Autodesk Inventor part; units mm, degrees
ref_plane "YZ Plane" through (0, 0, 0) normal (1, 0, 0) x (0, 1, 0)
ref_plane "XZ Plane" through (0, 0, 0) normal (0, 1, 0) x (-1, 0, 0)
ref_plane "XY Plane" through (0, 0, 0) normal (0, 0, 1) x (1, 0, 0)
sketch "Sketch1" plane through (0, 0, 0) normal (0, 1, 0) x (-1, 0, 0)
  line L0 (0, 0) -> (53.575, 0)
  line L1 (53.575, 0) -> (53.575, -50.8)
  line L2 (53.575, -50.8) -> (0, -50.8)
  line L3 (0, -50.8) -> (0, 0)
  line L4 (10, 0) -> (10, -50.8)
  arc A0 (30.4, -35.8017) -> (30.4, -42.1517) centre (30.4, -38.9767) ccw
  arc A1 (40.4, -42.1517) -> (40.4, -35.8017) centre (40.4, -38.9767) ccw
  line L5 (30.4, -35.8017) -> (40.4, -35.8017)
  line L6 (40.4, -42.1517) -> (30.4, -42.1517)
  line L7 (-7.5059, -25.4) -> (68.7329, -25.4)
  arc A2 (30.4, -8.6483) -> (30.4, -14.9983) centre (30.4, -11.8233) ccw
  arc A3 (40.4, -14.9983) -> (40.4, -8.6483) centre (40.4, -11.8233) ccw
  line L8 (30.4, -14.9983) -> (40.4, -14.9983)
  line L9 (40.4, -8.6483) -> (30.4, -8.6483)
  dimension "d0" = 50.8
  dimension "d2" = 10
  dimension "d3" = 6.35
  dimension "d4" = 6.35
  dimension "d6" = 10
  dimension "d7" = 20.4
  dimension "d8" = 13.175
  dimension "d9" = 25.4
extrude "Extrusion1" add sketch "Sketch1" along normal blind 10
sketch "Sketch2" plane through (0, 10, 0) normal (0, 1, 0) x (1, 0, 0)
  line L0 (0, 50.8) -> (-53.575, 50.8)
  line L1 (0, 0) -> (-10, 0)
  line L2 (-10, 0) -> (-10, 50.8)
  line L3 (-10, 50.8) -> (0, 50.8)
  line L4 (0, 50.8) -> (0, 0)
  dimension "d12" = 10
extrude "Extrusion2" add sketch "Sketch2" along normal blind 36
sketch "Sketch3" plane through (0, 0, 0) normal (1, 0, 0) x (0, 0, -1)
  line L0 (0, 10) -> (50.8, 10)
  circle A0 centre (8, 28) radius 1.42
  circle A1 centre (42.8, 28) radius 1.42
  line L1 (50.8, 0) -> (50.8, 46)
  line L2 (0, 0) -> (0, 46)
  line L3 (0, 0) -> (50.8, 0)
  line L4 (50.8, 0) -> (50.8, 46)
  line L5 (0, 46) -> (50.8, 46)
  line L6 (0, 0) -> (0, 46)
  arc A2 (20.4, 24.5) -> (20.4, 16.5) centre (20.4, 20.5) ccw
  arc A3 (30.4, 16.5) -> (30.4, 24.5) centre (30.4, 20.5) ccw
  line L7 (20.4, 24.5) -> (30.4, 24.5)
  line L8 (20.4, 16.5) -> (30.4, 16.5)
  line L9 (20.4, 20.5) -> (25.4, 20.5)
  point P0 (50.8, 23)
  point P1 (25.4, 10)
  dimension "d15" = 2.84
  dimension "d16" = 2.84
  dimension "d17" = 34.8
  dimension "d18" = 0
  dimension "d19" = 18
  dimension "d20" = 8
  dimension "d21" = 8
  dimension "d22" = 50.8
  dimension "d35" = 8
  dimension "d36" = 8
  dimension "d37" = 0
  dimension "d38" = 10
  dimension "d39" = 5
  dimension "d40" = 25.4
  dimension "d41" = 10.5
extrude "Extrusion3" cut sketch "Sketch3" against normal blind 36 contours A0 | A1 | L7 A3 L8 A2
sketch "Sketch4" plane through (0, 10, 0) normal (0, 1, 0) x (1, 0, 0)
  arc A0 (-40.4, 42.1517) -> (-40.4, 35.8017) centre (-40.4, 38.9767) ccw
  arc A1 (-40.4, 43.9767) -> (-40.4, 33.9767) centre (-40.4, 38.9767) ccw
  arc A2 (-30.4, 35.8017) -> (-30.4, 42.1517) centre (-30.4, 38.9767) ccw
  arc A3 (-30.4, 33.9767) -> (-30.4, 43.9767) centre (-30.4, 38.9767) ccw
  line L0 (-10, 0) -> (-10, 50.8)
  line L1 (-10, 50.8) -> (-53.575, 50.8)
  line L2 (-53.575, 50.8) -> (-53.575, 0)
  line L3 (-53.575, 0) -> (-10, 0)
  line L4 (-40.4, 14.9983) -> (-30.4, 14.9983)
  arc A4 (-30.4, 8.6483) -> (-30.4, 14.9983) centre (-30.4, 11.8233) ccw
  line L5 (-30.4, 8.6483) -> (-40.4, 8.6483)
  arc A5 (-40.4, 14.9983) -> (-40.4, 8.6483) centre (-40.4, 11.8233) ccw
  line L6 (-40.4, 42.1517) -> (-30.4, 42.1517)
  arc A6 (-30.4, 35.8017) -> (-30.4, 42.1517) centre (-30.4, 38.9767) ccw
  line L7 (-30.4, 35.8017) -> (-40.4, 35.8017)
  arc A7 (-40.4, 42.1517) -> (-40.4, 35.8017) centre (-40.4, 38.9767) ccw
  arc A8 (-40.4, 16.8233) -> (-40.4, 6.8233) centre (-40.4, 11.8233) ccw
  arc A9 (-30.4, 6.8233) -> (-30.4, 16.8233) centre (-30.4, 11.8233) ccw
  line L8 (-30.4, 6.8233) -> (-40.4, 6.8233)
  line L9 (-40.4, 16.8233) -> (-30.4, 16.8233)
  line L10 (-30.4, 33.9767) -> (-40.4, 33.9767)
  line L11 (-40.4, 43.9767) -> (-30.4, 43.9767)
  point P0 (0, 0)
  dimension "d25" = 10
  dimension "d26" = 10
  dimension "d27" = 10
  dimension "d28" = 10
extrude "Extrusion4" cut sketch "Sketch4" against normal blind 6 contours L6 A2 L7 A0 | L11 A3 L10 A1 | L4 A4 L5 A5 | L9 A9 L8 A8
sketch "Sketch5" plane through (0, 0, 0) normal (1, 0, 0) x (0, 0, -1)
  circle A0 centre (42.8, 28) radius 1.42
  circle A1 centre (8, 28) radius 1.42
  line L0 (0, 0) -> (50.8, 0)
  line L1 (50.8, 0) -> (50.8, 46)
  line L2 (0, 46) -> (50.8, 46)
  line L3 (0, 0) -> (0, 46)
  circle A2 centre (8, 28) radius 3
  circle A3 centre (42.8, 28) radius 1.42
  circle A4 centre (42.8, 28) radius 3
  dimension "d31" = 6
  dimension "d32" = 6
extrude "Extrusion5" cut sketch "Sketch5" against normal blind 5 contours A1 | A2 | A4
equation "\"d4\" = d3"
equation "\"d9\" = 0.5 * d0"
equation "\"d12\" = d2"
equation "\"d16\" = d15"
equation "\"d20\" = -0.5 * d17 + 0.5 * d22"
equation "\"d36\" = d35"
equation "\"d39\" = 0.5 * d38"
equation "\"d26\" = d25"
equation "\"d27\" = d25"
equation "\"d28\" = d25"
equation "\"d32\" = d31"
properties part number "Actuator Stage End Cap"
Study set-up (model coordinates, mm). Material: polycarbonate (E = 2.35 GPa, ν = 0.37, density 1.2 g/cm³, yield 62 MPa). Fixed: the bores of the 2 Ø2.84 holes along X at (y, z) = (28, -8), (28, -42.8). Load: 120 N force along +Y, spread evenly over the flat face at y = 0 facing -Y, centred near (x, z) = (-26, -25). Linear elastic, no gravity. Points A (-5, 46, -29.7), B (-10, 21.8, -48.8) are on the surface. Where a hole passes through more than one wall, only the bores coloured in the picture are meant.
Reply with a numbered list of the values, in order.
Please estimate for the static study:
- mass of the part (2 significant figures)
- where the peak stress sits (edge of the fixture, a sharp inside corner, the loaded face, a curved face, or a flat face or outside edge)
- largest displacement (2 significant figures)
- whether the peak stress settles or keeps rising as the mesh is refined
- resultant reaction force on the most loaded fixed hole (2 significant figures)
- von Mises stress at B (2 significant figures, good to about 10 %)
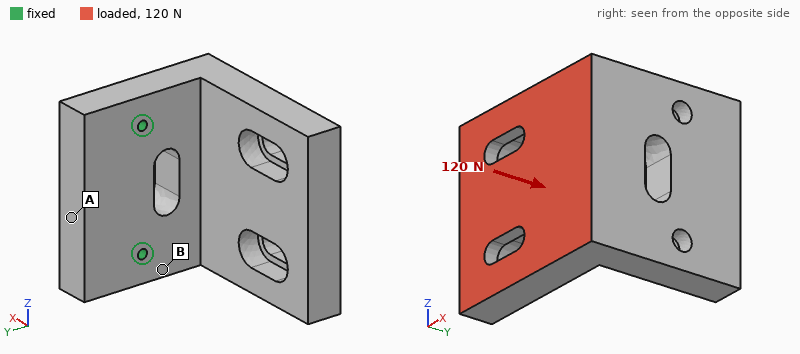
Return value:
1. 49 g
2. edge of the fixture
3. 0.90 mm
4. keeps rising
5. 62 N
6. 4.4 MPa
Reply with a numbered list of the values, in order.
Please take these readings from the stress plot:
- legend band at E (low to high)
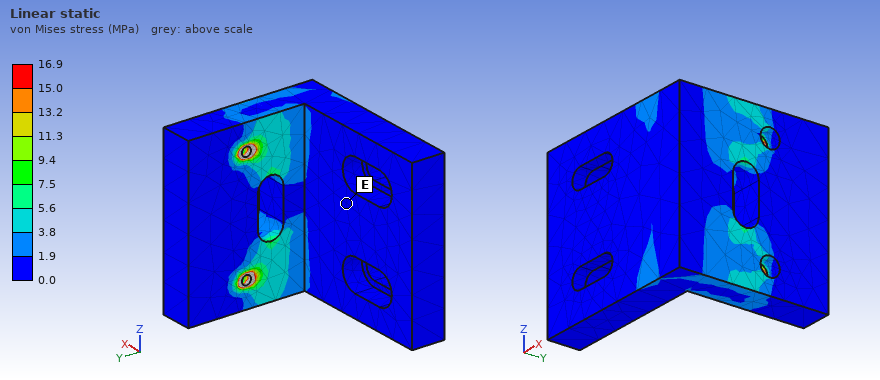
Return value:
1. 0.0 to 1.9 MPa
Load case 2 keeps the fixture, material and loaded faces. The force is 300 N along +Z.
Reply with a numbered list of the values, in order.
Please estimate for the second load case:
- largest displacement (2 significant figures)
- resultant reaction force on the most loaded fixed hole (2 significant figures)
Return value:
1. 0.46 mm
2. 320 N
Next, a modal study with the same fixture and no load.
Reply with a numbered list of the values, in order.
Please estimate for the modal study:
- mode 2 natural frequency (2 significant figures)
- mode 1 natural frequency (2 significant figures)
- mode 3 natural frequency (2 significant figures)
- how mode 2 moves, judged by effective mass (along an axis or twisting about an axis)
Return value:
1. 840 Hz
2. 360 Hz
3. 1200 Hz
4. along Z
